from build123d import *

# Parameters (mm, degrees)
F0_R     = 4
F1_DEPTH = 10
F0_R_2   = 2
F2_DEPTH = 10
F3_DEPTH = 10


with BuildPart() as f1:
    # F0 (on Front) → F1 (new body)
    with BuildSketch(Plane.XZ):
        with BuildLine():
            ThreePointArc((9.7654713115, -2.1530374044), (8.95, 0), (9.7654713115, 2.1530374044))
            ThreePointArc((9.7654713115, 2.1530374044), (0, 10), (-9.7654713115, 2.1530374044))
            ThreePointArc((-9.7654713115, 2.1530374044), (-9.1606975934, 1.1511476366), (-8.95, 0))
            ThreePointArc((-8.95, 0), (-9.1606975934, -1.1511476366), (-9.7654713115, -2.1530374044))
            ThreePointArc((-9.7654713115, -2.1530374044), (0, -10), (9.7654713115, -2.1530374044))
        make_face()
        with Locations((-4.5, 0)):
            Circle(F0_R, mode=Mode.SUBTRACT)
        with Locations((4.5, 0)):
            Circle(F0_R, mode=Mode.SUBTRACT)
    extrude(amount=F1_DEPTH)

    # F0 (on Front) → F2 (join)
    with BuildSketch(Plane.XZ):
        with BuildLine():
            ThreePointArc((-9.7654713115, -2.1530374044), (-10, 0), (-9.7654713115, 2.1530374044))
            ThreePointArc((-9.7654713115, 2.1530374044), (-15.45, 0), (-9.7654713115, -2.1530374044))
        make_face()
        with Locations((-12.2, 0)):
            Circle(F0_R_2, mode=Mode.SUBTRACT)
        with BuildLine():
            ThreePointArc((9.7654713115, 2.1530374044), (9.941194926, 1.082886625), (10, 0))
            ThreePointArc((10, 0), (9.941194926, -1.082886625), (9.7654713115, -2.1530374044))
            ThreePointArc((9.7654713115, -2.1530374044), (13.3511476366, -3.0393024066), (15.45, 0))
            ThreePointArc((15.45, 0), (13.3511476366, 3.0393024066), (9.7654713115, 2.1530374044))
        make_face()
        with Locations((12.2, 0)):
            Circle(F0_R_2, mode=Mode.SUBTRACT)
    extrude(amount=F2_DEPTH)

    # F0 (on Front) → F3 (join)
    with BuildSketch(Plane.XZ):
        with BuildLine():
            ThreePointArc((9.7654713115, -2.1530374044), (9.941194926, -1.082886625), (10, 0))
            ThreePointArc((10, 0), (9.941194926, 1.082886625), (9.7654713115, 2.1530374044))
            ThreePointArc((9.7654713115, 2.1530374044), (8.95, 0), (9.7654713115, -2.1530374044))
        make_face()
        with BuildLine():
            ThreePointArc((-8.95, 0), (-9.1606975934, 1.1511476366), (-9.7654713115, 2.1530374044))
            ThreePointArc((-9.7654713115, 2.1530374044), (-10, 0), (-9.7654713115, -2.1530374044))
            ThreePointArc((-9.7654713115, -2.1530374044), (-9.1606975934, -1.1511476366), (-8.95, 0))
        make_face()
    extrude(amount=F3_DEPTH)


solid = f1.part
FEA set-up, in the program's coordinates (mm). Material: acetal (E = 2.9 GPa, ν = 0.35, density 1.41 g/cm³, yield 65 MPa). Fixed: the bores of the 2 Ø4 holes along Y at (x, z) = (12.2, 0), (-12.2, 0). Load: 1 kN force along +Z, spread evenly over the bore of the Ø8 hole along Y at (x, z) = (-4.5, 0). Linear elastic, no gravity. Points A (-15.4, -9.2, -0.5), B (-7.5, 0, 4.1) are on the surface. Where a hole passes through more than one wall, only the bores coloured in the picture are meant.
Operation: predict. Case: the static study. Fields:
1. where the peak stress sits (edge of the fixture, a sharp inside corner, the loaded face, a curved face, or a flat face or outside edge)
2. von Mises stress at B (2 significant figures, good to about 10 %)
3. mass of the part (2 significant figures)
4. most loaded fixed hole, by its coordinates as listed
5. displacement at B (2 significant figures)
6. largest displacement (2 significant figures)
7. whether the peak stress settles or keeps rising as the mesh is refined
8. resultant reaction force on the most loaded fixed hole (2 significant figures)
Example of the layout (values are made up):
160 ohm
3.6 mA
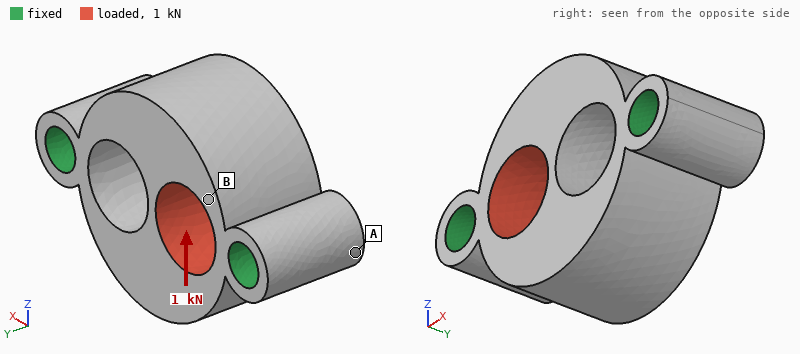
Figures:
edge of the fixture
11 MPa
3.5 g
(-12.2, 0)
49 µm
70 µm
keeps rising
740 N
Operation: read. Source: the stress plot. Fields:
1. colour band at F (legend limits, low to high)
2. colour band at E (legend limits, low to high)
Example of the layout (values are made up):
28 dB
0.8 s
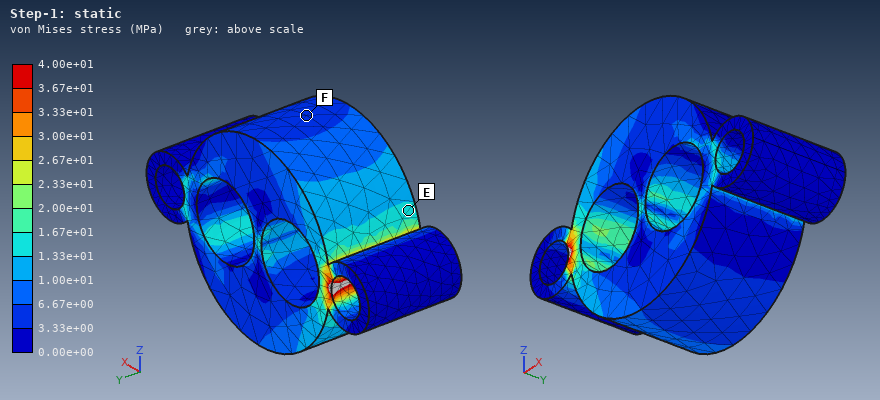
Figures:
3.33e+00 to 6.67e+00 MPa
1.33e+01 to 1.67e+01 MPa
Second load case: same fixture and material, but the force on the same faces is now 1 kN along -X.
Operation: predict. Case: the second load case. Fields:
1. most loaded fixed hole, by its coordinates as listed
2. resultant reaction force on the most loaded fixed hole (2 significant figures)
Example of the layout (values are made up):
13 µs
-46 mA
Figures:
(-12.2, 0)
660 N
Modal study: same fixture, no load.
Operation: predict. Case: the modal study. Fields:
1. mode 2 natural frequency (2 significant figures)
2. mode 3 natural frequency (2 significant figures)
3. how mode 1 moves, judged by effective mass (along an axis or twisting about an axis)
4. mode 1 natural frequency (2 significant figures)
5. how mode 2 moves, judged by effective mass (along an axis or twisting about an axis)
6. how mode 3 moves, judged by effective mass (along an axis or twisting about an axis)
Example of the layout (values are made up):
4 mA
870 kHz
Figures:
8700 Hz
10 kHz
twisting about X
7600 Hz
along Y
along X
